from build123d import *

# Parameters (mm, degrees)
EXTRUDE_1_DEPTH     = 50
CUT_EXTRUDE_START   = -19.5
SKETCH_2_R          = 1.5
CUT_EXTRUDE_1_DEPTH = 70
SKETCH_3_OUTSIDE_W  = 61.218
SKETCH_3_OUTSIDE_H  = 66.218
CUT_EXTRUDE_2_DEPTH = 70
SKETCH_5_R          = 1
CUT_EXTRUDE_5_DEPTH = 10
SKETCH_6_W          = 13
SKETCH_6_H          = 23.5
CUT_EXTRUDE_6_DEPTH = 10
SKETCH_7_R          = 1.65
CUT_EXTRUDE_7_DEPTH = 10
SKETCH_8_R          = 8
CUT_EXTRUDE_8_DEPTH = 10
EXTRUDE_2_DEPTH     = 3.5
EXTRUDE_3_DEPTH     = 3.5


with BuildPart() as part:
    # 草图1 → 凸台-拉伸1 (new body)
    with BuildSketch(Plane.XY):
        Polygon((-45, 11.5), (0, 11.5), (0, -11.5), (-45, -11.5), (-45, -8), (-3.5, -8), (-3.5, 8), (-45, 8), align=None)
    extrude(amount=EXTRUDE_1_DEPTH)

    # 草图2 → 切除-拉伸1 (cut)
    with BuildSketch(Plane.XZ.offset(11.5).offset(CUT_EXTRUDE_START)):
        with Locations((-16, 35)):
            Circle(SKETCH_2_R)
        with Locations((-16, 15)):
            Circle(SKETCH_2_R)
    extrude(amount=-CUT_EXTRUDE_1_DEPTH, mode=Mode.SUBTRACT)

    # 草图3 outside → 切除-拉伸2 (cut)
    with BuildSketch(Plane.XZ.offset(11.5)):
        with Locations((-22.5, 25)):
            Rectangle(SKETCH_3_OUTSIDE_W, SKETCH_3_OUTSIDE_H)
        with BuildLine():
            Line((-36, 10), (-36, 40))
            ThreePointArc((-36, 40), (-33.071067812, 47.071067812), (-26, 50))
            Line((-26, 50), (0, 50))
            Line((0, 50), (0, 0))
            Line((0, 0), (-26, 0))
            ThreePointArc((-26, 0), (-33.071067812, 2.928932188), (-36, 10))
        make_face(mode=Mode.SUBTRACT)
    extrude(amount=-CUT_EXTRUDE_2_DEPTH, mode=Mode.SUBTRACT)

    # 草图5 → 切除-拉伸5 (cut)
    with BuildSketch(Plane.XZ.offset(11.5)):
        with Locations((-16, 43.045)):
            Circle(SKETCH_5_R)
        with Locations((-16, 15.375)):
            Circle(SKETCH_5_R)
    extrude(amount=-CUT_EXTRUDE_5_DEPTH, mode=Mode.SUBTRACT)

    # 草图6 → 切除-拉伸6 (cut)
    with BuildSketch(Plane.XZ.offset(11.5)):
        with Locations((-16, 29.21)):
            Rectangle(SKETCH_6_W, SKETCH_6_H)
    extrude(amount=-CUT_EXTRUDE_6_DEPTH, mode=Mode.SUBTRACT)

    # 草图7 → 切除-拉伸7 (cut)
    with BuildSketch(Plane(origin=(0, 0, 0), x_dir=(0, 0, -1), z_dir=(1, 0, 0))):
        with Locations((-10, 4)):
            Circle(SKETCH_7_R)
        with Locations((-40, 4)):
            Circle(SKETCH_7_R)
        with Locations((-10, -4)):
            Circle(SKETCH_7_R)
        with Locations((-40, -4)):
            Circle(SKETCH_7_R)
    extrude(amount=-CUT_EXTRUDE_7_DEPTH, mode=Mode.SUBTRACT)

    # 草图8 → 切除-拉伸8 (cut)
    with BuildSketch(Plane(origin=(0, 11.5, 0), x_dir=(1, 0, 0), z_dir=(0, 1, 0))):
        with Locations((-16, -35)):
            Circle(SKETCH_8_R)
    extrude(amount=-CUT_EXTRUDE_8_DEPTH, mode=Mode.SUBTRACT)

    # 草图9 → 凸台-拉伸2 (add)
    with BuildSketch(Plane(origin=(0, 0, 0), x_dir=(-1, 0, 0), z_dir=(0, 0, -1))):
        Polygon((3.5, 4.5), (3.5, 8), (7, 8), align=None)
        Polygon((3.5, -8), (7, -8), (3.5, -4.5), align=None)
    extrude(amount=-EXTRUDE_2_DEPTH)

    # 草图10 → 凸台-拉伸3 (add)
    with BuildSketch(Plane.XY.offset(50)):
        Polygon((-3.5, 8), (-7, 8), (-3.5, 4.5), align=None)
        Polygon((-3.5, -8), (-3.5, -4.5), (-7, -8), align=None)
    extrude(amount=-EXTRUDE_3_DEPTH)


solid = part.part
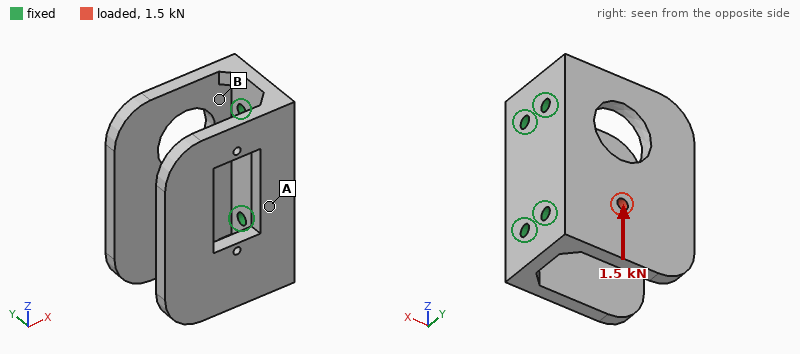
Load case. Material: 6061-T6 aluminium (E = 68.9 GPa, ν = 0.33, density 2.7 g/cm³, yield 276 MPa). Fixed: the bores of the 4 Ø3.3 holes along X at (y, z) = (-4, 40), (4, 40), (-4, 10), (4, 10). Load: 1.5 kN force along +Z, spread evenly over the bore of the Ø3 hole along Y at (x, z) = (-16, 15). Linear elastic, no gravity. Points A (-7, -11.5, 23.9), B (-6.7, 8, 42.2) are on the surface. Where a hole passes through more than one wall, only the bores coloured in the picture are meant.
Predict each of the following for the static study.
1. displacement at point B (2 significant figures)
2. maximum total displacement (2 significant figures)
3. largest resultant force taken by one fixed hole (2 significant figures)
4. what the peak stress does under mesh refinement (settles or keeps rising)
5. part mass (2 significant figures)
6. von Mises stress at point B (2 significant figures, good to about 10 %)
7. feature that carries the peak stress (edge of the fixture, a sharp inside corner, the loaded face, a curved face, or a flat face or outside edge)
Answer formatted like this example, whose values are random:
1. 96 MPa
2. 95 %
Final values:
1. 12 µm
2. 54 µm
3. 1.0 kN
4. keeps rising
5. 36 g
6. 14 MPa
7. edge of the fixture
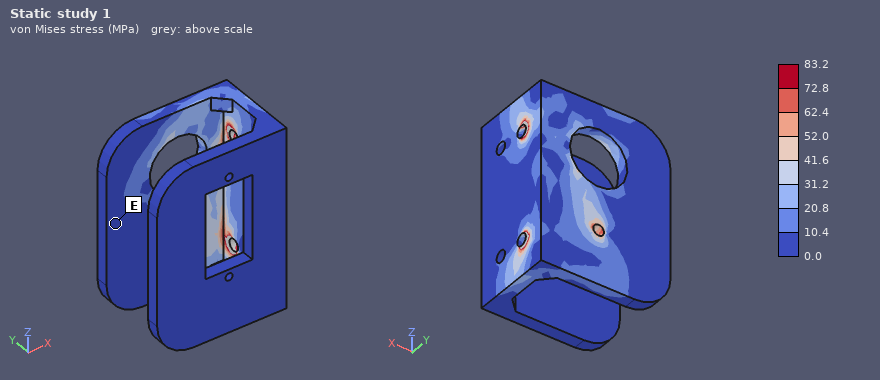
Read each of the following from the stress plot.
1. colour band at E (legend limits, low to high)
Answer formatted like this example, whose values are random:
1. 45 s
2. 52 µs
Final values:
1. 0.0 to 10.4 MPa
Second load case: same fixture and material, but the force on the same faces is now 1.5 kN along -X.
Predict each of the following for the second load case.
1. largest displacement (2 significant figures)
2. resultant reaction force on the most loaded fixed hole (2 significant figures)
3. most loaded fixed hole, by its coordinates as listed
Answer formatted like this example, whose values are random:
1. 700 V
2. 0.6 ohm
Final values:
1. 0.11 mm
2. 1.4 kN
3. (4, 10)
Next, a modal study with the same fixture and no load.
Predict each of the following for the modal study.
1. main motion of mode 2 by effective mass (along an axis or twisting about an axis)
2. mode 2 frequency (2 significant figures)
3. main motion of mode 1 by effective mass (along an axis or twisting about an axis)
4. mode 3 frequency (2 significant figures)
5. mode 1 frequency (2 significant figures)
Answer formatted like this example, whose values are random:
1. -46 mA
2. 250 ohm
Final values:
1. along Y
2. 2000 Hz
3. along Y
4. 4000 Hz
5. 1800 Hz
